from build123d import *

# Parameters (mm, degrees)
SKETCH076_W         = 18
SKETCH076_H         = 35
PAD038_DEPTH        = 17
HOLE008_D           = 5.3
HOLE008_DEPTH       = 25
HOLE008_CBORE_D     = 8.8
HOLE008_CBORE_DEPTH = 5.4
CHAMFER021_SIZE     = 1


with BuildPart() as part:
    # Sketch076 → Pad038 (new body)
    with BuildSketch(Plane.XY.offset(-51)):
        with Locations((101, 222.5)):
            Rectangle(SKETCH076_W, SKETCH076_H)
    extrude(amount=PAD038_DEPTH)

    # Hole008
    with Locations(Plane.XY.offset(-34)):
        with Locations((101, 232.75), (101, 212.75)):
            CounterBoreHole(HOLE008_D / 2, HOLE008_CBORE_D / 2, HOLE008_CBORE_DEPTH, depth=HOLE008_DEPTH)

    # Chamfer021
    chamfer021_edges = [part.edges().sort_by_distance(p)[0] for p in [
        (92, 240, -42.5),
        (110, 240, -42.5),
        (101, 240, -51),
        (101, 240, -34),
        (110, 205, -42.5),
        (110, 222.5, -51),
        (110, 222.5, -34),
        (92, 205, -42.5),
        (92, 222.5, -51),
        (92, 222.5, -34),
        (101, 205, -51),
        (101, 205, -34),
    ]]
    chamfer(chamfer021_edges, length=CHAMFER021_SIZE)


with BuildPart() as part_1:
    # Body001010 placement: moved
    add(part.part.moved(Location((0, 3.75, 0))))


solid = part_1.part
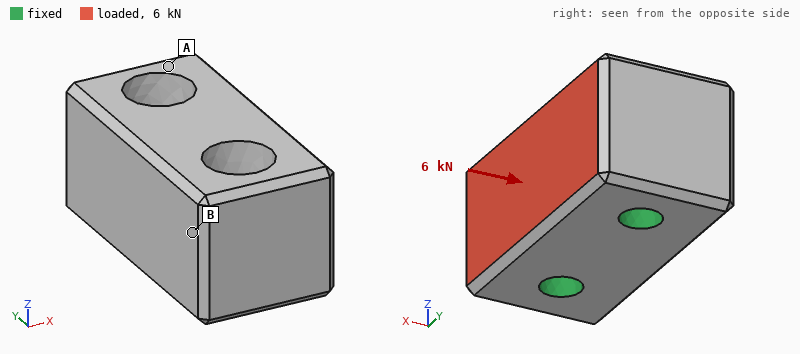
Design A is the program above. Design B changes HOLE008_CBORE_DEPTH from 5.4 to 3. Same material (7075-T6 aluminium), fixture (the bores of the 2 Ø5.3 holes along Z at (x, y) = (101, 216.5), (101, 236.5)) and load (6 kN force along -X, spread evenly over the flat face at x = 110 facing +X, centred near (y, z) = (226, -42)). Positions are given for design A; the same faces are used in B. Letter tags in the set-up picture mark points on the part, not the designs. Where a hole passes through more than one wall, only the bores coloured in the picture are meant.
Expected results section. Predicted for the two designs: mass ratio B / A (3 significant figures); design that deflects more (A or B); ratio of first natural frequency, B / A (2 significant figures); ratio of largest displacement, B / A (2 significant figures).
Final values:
1.02
A
1.3
0.53
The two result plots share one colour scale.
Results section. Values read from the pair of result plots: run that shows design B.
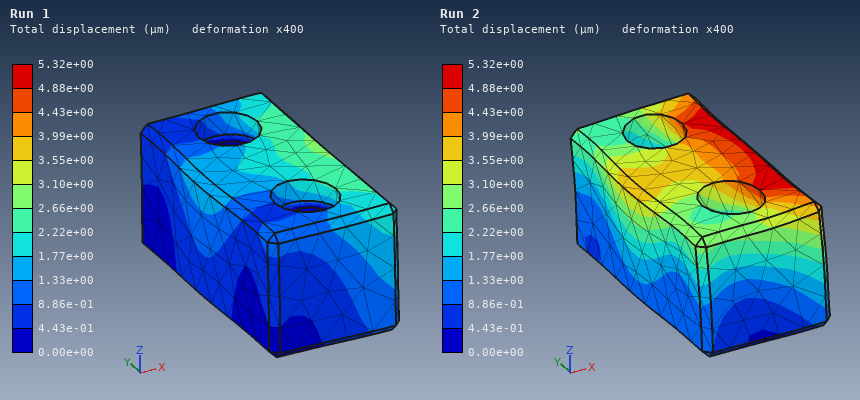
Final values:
Run 1
